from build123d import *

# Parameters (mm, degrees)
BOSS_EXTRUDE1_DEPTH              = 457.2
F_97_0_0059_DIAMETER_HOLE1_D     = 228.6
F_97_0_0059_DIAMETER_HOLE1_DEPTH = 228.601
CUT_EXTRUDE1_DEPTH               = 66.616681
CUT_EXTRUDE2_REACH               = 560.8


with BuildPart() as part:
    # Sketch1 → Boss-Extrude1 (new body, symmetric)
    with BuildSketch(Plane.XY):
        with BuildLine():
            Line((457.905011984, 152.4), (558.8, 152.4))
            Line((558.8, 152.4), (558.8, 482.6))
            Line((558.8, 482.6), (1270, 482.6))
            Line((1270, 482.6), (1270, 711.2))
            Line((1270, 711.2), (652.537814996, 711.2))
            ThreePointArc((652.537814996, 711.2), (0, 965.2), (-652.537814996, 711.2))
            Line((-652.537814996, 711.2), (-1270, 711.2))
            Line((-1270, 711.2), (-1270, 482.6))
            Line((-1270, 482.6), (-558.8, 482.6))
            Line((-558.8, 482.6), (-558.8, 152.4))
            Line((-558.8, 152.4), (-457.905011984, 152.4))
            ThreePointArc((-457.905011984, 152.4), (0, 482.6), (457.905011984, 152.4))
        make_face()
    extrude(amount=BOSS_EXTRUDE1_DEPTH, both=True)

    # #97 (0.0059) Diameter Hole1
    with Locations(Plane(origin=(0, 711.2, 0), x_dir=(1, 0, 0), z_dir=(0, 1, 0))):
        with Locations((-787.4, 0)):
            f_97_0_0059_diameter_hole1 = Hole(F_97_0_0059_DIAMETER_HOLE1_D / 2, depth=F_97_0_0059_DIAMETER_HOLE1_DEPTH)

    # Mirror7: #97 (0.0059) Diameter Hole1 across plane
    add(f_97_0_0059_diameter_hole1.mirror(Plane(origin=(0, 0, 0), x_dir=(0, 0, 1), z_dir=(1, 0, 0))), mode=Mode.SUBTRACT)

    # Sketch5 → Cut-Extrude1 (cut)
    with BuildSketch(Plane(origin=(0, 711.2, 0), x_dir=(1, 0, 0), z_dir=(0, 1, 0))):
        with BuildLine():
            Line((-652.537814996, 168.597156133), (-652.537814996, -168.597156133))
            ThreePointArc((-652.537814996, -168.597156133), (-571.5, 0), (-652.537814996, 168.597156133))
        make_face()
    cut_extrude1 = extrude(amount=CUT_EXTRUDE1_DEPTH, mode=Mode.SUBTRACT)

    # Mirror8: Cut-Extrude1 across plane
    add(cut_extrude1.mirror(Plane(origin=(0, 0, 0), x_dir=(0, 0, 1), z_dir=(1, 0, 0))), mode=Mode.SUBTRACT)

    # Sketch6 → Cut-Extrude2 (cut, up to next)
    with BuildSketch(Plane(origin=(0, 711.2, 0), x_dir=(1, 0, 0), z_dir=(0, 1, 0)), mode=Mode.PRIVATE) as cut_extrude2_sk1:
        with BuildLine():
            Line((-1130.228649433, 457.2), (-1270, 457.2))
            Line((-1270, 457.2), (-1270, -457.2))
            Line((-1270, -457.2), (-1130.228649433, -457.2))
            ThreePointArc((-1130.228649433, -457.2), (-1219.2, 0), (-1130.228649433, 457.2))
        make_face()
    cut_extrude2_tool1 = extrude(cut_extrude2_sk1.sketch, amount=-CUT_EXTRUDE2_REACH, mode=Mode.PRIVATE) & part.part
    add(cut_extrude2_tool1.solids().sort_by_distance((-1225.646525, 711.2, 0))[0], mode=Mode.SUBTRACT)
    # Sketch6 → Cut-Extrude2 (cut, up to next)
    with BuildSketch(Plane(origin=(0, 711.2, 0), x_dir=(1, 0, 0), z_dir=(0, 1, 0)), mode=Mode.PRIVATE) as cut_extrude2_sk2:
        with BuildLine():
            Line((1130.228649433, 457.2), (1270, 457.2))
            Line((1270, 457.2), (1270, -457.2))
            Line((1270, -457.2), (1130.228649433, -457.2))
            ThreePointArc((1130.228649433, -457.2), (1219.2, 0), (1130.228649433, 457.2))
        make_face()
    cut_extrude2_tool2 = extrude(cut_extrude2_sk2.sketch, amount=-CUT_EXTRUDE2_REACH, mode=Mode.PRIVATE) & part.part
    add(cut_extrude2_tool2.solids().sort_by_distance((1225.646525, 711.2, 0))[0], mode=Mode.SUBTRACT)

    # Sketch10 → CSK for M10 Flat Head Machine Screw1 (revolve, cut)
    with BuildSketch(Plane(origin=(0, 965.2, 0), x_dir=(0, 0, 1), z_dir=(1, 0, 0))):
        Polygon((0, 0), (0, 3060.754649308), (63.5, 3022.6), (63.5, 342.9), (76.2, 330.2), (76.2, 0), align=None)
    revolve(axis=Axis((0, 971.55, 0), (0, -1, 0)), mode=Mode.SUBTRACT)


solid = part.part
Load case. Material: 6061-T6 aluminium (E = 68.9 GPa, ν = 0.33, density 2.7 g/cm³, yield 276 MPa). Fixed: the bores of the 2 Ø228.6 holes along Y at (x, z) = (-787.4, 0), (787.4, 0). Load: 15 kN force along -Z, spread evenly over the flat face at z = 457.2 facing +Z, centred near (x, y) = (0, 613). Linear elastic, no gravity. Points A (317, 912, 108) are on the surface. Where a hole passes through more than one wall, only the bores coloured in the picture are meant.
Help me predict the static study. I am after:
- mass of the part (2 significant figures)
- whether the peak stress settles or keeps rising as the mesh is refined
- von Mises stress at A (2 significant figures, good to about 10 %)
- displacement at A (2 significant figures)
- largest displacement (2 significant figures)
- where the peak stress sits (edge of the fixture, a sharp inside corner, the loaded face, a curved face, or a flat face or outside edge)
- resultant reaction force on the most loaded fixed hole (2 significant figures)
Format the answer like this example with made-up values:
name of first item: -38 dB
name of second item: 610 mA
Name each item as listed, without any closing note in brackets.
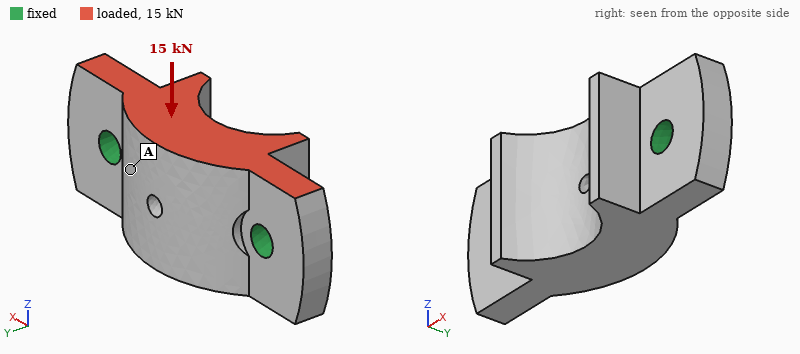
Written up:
mass of the part: 2200 kg
whether the peak stress settles or keeps rising as the mesh is refined: keeps rising
von Mises stress at A: 0.022 MPa
displacement at A: 0.67 µm
largest displacement: 0.90 µm
where the peak stress sits: edge of the fixture
resultant reaction force on the most loaded fixed hole: 7.5 kN
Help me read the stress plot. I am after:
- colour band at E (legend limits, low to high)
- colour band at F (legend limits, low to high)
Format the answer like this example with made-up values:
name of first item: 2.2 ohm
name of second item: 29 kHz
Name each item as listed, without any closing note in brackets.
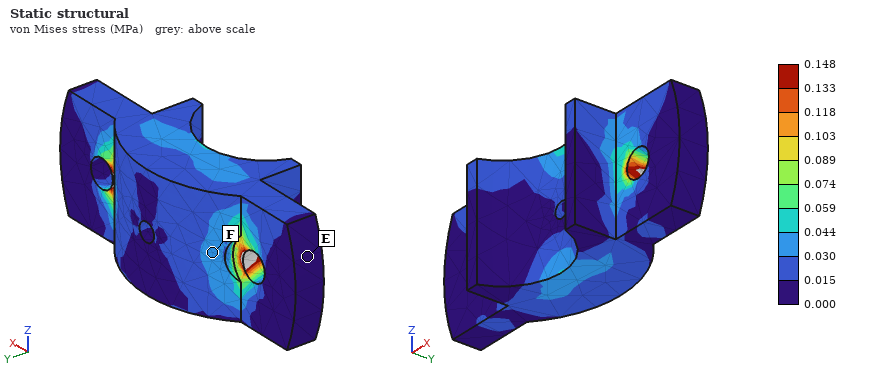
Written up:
colour band at E: 0.000 to 0.015 MPa
colour band at F: 0.030 to 0.044 MPa
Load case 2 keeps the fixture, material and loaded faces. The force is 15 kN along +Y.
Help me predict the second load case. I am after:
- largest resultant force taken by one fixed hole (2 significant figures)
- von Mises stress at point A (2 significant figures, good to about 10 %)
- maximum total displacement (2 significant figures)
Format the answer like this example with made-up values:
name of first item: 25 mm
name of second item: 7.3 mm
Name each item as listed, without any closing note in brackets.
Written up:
largest resultant force taken by one fixed hole: 7.8 kN
von Mises stress at point A: 0.074 MPa
maximum total displacement: 5.4 µm
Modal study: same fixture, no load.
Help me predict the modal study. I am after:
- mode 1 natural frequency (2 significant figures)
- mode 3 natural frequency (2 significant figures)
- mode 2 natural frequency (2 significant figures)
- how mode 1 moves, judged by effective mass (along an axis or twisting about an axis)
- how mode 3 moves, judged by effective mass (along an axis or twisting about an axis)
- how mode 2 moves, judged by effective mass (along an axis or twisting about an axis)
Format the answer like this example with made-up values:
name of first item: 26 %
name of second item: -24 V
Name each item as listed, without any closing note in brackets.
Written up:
mode 1 natural frequency: 350 Hz
mode 3 natural frequency: 580 Hz
mode 2 natural frequency: 450 Hz
how mode 1 moves, judged by effective mass: twisting about X
how mode 3 moves, judged by effective mass: along Z
how mode 2 moves, judged by effective mass: along Y
